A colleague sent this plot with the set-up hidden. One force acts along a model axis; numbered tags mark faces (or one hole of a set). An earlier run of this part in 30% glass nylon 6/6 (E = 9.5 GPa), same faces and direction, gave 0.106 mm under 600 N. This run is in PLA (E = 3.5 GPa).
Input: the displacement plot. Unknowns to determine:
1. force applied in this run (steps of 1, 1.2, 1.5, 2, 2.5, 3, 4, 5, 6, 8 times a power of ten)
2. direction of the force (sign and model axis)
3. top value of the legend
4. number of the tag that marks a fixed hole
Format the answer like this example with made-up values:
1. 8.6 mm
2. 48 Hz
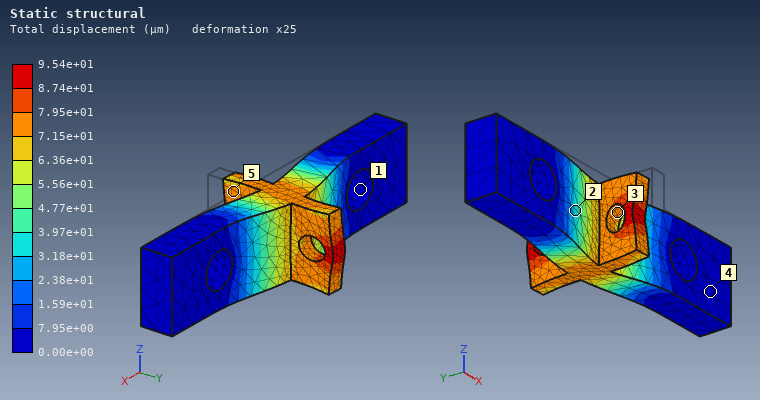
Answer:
1. 200 N
2. +Y
3. 9.54e+01 µm
4. 1
